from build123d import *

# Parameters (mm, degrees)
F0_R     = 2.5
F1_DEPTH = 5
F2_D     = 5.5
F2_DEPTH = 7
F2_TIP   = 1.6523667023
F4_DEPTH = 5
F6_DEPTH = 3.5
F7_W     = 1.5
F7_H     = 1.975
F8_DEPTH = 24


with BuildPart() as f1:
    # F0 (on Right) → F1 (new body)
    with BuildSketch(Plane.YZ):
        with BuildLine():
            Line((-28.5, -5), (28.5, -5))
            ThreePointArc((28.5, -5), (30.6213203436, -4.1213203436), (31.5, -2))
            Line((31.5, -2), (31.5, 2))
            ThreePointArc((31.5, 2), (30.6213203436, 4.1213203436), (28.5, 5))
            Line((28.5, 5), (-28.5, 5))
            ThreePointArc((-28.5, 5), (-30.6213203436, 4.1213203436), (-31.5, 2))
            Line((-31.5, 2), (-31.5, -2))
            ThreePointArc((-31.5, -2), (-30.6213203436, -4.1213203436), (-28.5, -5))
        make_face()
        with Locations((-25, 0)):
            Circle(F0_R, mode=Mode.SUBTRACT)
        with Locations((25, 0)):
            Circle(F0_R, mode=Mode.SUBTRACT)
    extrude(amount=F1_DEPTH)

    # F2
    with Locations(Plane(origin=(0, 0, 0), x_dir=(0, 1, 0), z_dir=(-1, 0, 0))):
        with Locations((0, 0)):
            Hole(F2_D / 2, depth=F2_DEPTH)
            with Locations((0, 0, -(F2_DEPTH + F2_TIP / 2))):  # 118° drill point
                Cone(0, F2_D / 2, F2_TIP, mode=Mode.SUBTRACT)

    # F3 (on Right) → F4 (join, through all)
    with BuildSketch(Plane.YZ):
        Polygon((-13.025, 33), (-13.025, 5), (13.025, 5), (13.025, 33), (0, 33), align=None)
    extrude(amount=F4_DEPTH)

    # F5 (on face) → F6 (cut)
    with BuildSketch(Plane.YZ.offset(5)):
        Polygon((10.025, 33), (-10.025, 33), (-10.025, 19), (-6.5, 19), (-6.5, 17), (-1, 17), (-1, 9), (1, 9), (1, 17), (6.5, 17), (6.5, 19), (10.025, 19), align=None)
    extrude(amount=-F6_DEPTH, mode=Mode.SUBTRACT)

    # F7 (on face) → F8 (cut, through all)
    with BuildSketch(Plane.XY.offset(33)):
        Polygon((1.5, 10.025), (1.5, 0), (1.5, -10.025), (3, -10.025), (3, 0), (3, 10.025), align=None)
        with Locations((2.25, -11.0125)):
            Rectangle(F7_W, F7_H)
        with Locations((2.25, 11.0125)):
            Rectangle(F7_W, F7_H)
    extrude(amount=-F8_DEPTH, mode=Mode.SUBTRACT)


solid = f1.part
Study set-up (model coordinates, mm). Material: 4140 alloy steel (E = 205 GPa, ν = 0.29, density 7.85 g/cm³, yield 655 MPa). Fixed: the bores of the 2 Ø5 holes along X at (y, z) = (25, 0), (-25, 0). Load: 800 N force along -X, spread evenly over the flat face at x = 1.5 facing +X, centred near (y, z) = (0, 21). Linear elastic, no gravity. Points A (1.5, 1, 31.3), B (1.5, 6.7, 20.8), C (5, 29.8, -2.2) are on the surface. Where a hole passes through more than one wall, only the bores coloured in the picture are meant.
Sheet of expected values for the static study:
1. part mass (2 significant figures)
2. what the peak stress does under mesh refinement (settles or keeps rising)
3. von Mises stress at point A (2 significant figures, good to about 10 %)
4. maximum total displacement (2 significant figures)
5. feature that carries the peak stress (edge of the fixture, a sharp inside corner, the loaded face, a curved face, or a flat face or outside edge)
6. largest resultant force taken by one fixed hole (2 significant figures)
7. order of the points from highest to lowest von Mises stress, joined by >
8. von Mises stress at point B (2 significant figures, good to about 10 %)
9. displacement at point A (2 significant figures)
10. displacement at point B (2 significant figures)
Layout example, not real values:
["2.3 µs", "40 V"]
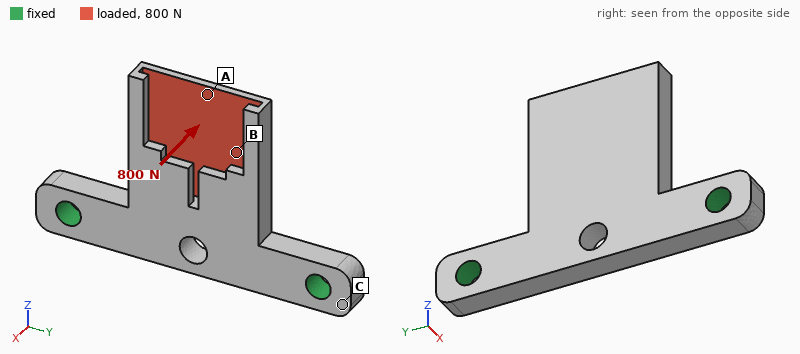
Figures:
["39 g", "keeps rising", "150 MPa", "0.37 mm", "a sharp inside corner", "420 N", "A > B > C", "97 MPa", "0.34 mm", "0.19 mm"]
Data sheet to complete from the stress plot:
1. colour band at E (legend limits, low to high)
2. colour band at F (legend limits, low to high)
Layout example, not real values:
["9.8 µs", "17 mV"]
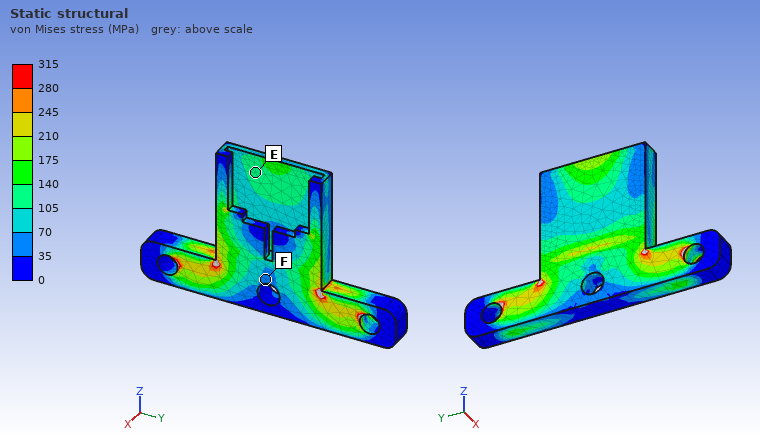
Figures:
["105 to 140 MPa", "35 to 70 MPa"]
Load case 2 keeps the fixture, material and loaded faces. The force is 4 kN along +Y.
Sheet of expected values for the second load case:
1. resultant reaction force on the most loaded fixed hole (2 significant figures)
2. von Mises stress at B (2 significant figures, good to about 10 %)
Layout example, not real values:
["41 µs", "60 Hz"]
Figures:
["2.9 kN", "140 MPa"]
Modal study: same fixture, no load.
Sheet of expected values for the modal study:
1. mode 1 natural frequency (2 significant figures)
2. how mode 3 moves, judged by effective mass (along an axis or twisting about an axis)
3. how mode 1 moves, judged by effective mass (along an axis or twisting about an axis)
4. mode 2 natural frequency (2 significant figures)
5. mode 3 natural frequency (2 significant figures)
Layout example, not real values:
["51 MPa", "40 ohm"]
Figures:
["2900 Hz", "along X", "along X", "6500 Hz", "9200 Hz"]
